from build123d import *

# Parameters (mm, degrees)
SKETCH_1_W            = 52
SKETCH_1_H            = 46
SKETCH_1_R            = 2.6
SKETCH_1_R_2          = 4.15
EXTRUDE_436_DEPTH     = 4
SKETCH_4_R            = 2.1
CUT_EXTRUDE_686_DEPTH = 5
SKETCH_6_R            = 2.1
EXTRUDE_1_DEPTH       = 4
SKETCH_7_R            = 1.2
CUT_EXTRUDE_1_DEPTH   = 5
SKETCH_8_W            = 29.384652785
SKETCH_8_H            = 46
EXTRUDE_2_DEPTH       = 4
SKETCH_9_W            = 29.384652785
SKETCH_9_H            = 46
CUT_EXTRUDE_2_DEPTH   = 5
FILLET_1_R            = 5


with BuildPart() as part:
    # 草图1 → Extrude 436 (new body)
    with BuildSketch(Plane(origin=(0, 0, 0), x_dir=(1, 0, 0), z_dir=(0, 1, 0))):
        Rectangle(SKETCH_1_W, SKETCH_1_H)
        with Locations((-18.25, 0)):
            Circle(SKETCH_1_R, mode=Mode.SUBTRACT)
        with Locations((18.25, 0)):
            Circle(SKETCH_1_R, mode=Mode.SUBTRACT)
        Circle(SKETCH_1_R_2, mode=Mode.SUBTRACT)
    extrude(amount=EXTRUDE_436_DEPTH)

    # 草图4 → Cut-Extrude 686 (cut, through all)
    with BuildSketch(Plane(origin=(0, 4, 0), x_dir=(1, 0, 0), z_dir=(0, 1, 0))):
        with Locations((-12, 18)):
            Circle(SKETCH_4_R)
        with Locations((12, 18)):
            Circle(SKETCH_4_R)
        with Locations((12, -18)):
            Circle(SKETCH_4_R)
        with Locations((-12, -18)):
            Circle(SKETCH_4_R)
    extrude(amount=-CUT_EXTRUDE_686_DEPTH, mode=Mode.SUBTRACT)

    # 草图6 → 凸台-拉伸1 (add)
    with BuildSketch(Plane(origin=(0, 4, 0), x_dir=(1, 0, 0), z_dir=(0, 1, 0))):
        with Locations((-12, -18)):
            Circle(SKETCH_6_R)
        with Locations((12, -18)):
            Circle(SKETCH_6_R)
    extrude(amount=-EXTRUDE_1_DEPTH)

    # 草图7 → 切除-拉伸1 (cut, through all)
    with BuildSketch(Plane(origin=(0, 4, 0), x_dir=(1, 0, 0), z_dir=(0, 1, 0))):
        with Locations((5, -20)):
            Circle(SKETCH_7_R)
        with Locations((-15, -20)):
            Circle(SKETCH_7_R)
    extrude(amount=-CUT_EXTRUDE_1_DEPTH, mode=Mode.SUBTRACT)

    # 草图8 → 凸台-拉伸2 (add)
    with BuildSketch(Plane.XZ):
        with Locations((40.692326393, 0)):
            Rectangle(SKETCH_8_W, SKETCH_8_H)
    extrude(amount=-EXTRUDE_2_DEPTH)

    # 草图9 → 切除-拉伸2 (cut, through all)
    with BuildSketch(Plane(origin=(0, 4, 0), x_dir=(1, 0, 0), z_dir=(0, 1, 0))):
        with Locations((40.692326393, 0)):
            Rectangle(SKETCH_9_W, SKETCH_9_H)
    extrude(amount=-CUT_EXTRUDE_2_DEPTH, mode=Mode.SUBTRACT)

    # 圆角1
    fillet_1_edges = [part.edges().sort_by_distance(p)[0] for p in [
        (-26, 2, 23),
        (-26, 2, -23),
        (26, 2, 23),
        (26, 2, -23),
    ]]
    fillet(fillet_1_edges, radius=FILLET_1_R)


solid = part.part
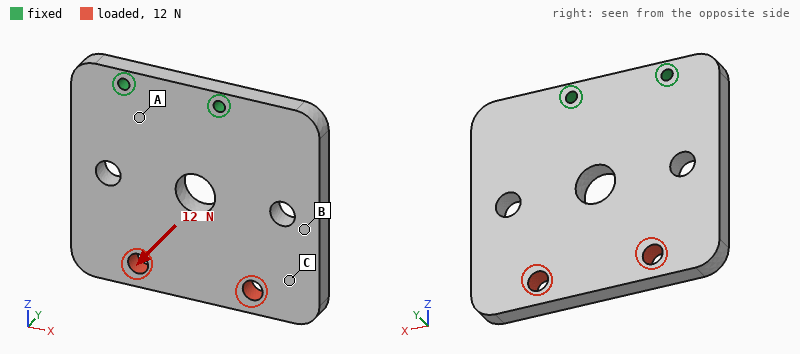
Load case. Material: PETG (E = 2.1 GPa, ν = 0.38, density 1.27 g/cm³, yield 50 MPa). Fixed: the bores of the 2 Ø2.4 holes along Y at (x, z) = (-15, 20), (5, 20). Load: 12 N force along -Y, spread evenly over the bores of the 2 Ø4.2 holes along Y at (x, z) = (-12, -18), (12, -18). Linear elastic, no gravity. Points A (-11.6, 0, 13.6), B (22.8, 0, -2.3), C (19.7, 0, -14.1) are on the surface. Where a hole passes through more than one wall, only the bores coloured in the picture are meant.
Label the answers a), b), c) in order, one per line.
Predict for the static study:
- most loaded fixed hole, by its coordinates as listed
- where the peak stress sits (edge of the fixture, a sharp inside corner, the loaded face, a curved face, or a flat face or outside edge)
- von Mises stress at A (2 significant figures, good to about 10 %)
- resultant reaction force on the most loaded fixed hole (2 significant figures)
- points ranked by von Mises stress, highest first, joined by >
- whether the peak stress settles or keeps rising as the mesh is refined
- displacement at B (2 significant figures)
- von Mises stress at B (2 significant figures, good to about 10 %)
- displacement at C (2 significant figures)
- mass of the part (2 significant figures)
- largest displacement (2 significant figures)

a) (5, 20)
b) edge of the fixture
c) 3.0 MPa
d) 8.5 N
e) A > B > C
f) keeps rising
g) 0.27 mm
h) 1.6 MPa
i) 0.49 mm
j) 11 g
k) 0.68 mm
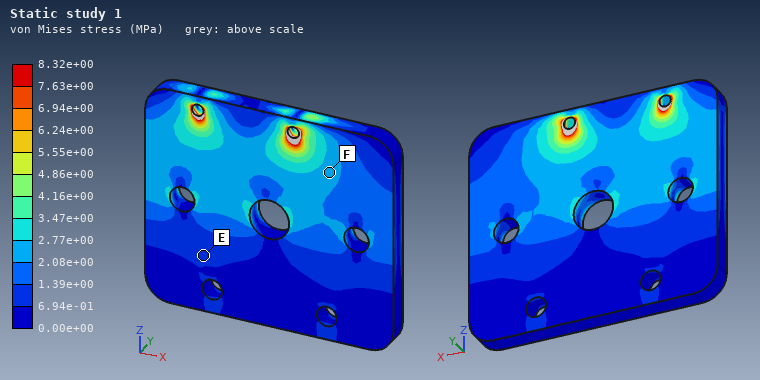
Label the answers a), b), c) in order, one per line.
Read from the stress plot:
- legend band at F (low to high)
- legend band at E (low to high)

a) 2.08e+00 to 2.77e+00 MPa
b) 6.94e-01 to 1.39e+00 MPa
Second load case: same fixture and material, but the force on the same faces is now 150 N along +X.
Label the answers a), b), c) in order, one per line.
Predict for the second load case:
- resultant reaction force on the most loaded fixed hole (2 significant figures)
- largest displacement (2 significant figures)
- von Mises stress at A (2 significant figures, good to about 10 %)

a) 270 N
b) 0.30 mm
c) 5.6 MPa
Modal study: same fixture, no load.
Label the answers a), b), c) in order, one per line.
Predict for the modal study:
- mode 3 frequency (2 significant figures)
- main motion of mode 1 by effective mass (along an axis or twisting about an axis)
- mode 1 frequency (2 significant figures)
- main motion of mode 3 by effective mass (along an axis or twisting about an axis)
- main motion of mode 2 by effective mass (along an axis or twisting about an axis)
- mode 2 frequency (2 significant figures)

a) 1700 Hz
b) along Y
c) 380 Hz
d) along X
e) twisting about Z
f) 730 Hz
